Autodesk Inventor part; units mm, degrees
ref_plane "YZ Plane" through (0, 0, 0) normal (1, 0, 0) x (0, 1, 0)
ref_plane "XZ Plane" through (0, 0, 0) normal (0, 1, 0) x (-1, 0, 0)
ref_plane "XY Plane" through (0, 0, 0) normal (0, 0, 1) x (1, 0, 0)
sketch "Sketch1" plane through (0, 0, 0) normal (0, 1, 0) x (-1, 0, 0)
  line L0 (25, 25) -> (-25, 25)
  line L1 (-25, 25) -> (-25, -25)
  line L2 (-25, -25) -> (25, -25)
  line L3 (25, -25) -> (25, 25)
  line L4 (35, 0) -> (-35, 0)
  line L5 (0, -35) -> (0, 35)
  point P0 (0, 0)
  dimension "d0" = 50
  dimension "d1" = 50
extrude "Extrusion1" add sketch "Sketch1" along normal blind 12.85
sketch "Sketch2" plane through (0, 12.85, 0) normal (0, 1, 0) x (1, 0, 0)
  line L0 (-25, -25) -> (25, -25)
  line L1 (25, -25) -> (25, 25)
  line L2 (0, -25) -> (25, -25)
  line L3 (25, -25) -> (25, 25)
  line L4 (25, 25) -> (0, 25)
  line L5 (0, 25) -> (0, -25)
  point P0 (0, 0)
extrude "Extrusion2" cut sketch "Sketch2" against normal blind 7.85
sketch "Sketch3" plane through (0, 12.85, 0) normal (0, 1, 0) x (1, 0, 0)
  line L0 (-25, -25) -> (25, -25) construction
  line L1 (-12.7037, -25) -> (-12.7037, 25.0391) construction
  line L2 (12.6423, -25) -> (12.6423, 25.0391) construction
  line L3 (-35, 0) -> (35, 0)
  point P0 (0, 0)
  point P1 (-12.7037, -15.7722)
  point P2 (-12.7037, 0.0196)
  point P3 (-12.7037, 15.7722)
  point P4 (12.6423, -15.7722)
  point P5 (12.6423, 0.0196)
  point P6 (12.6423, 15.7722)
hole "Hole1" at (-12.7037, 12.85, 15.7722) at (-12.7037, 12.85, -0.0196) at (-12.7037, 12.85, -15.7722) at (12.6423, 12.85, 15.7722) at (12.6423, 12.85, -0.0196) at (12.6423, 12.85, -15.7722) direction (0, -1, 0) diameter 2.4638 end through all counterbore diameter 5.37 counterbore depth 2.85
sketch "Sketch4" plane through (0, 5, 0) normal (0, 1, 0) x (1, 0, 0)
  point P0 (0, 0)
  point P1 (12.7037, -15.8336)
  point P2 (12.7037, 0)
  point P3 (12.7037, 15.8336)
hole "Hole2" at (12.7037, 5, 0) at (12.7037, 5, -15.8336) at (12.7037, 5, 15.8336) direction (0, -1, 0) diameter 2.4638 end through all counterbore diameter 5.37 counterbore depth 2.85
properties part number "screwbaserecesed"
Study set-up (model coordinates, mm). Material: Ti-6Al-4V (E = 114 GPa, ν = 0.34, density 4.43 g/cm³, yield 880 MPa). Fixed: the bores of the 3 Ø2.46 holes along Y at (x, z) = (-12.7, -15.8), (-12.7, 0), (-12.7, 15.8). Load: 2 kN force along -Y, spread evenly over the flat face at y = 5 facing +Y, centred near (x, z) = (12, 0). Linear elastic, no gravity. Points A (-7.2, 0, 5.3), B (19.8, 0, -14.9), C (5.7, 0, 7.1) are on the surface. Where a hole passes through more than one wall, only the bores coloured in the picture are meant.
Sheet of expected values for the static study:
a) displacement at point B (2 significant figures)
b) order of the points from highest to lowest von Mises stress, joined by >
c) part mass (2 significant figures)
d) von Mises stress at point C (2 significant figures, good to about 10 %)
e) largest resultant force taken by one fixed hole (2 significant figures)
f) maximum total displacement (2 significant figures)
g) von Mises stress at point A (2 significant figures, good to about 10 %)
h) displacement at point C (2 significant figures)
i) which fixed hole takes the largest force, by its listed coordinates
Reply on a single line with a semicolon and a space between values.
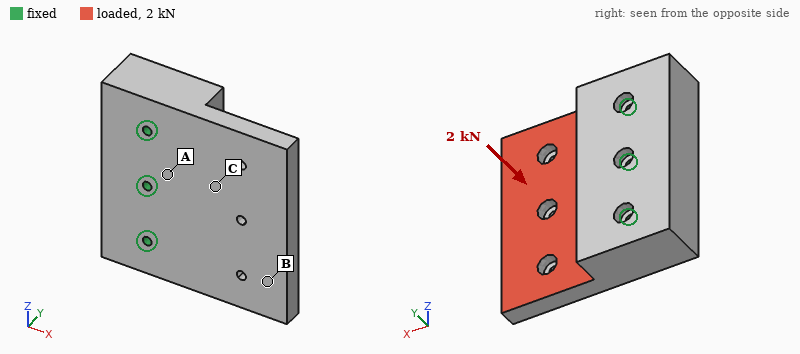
0.097 mm; C > A > B; 96 g; 66 MPa; 840 N; 0.13 mm; 34 MPa; 0.031 mm; (-12.7, 0)
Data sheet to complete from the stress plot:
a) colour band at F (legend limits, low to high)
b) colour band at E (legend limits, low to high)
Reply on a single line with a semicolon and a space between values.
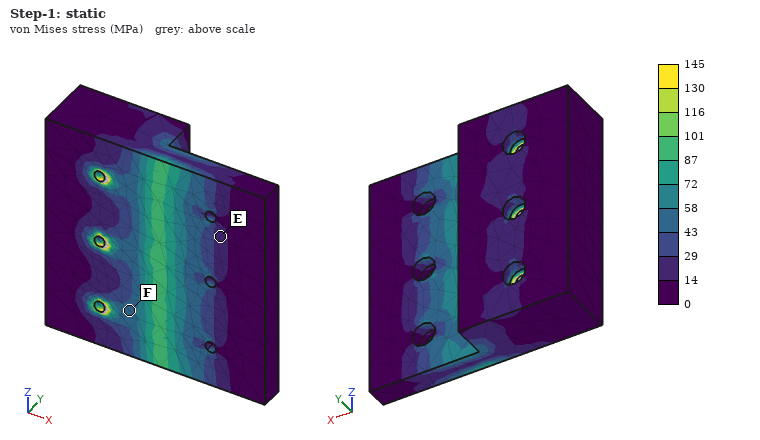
43 to 58 MPa; 14 to 29 MPa
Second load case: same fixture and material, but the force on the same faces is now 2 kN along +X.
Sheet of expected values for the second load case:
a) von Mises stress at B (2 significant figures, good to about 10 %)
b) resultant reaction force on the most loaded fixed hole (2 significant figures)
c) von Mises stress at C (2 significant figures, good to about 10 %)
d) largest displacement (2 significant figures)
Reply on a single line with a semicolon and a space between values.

3.4 MPa; 720 N; 11 MPa; 22 µm
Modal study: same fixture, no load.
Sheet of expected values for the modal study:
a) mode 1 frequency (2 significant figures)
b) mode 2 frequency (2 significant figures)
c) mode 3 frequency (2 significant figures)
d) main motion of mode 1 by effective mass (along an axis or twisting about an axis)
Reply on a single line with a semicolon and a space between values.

4800 Hz; 7600 Hz; 15 kHz; along Y
